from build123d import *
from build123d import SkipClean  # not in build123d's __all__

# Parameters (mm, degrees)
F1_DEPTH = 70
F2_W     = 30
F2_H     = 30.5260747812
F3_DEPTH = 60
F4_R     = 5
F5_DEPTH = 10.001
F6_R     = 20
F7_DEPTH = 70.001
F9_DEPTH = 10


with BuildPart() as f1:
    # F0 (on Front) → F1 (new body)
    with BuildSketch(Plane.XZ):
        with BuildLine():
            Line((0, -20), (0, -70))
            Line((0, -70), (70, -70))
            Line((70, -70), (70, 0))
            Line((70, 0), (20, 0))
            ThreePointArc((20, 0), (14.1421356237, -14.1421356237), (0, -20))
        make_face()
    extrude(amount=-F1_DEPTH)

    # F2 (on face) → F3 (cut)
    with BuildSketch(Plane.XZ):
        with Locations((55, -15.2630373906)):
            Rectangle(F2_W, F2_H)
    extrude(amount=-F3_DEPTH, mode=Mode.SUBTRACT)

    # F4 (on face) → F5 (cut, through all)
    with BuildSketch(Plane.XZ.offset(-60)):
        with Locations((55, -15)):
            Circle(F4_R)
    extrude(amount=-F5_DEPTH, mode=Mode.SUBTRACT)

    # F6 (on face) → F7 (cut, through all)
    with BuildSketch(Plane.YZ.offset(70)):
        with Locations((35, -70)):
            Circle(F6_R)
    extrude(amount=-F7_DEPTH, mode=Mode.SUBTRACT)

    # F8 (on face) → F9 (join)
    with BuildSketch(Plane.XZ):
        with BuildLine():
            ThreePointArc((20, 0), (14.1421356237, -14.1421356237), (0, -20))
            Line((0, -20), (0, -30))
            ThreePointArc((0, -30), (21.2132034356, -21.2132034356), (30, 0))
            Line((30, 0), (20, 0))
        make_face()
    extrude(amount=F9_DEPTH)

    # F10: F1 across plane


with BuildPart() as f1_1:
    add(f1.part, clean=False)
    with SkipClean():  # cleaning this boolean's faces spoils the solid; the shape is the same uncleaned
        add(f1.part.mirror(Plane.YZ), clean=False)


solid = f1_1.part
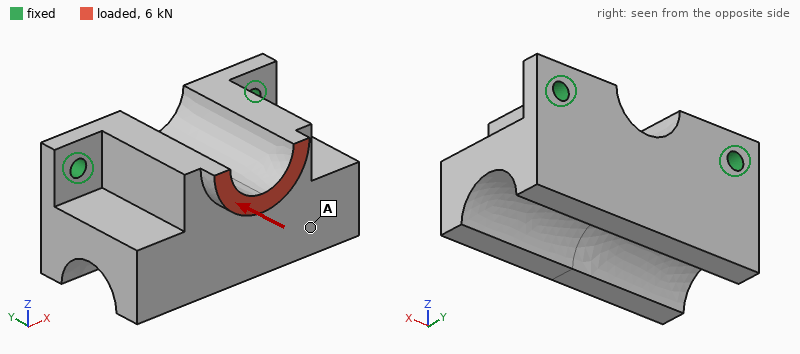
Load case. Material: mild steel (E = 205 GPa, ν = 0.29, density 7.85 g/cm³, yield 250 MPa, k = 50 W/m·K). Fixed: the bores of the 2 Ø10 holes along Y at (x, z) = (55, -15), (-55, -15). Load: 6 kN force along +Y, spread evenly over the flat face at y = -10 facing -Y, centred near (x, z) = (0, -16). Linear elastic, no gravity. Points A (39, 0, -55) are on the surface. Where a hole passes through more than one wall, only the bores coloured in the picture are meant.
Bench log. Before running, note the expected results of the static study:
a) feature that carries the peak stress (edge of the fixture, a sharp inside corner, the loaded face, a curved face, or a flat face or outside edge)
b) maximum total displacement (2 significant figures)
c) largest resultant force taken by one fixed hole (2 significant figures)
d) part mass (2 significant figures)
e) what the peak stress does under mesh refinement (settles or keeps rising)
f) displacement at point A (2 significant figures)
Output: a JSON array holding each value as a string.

["edge of the fixture", "12 µm", "3.1 kN", "3.5 kg", "keeps rising", "6.9 µm"]
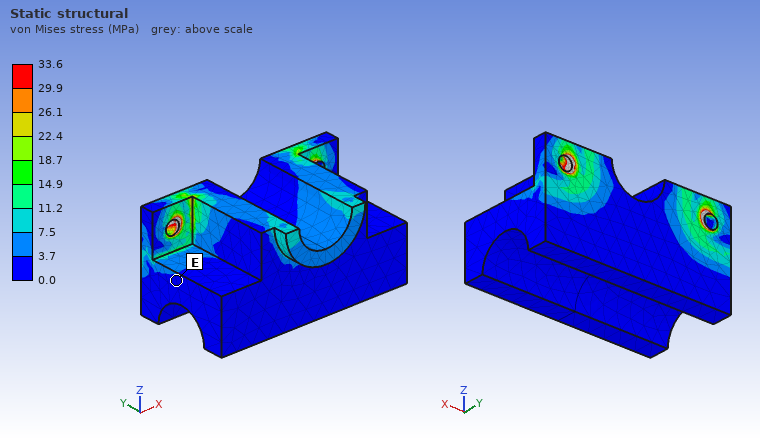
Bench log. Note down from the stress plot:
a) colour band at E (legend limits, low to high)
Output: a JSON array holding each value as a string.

["0.0 to 3.7 MPa"]
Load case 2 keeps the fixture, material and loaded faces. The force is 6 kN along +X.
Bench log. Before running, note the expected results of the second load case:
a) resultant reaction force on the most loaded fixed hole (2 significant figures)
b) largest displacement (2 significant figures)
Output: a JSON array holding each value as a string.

["5.3 kN", "19 µm"]
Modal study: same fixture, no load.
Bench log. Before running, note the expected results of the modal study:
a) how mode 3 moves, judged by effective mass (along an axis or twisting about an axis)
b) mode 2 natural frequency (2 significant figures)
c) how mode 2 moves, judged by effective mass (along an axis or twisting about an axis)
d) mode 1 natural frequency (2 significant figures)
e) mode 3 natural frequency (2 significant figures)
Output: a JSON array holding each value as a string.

["along Y", "3200 Hz", "along X", "790 Hz", "3800 Hz"]
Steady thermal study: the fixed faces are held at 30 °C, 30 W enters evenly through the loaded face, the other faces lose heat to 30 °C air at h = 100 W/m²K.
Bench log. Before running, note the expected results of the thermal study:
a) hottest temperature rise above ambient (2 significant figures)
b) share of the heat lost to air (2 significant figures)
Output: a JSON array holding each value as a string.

["20 K", "77 %"]
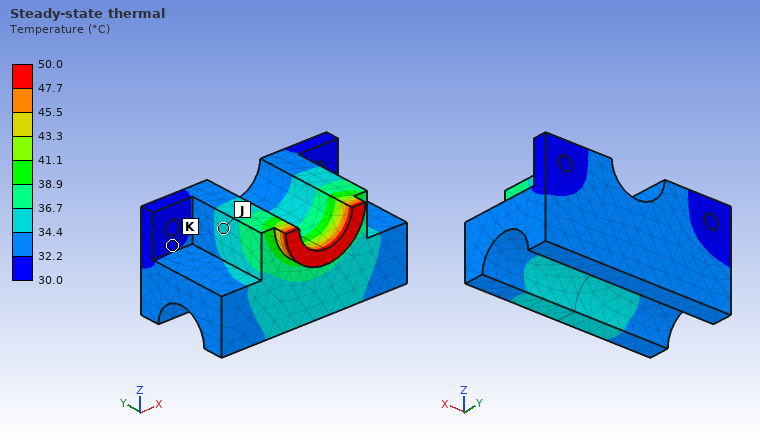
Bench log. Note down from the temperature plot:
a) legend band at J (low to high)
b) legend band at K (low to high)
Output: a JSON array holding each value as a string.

["34.4 to 36.7 °C", "30.0 to 32.2 °C"]
